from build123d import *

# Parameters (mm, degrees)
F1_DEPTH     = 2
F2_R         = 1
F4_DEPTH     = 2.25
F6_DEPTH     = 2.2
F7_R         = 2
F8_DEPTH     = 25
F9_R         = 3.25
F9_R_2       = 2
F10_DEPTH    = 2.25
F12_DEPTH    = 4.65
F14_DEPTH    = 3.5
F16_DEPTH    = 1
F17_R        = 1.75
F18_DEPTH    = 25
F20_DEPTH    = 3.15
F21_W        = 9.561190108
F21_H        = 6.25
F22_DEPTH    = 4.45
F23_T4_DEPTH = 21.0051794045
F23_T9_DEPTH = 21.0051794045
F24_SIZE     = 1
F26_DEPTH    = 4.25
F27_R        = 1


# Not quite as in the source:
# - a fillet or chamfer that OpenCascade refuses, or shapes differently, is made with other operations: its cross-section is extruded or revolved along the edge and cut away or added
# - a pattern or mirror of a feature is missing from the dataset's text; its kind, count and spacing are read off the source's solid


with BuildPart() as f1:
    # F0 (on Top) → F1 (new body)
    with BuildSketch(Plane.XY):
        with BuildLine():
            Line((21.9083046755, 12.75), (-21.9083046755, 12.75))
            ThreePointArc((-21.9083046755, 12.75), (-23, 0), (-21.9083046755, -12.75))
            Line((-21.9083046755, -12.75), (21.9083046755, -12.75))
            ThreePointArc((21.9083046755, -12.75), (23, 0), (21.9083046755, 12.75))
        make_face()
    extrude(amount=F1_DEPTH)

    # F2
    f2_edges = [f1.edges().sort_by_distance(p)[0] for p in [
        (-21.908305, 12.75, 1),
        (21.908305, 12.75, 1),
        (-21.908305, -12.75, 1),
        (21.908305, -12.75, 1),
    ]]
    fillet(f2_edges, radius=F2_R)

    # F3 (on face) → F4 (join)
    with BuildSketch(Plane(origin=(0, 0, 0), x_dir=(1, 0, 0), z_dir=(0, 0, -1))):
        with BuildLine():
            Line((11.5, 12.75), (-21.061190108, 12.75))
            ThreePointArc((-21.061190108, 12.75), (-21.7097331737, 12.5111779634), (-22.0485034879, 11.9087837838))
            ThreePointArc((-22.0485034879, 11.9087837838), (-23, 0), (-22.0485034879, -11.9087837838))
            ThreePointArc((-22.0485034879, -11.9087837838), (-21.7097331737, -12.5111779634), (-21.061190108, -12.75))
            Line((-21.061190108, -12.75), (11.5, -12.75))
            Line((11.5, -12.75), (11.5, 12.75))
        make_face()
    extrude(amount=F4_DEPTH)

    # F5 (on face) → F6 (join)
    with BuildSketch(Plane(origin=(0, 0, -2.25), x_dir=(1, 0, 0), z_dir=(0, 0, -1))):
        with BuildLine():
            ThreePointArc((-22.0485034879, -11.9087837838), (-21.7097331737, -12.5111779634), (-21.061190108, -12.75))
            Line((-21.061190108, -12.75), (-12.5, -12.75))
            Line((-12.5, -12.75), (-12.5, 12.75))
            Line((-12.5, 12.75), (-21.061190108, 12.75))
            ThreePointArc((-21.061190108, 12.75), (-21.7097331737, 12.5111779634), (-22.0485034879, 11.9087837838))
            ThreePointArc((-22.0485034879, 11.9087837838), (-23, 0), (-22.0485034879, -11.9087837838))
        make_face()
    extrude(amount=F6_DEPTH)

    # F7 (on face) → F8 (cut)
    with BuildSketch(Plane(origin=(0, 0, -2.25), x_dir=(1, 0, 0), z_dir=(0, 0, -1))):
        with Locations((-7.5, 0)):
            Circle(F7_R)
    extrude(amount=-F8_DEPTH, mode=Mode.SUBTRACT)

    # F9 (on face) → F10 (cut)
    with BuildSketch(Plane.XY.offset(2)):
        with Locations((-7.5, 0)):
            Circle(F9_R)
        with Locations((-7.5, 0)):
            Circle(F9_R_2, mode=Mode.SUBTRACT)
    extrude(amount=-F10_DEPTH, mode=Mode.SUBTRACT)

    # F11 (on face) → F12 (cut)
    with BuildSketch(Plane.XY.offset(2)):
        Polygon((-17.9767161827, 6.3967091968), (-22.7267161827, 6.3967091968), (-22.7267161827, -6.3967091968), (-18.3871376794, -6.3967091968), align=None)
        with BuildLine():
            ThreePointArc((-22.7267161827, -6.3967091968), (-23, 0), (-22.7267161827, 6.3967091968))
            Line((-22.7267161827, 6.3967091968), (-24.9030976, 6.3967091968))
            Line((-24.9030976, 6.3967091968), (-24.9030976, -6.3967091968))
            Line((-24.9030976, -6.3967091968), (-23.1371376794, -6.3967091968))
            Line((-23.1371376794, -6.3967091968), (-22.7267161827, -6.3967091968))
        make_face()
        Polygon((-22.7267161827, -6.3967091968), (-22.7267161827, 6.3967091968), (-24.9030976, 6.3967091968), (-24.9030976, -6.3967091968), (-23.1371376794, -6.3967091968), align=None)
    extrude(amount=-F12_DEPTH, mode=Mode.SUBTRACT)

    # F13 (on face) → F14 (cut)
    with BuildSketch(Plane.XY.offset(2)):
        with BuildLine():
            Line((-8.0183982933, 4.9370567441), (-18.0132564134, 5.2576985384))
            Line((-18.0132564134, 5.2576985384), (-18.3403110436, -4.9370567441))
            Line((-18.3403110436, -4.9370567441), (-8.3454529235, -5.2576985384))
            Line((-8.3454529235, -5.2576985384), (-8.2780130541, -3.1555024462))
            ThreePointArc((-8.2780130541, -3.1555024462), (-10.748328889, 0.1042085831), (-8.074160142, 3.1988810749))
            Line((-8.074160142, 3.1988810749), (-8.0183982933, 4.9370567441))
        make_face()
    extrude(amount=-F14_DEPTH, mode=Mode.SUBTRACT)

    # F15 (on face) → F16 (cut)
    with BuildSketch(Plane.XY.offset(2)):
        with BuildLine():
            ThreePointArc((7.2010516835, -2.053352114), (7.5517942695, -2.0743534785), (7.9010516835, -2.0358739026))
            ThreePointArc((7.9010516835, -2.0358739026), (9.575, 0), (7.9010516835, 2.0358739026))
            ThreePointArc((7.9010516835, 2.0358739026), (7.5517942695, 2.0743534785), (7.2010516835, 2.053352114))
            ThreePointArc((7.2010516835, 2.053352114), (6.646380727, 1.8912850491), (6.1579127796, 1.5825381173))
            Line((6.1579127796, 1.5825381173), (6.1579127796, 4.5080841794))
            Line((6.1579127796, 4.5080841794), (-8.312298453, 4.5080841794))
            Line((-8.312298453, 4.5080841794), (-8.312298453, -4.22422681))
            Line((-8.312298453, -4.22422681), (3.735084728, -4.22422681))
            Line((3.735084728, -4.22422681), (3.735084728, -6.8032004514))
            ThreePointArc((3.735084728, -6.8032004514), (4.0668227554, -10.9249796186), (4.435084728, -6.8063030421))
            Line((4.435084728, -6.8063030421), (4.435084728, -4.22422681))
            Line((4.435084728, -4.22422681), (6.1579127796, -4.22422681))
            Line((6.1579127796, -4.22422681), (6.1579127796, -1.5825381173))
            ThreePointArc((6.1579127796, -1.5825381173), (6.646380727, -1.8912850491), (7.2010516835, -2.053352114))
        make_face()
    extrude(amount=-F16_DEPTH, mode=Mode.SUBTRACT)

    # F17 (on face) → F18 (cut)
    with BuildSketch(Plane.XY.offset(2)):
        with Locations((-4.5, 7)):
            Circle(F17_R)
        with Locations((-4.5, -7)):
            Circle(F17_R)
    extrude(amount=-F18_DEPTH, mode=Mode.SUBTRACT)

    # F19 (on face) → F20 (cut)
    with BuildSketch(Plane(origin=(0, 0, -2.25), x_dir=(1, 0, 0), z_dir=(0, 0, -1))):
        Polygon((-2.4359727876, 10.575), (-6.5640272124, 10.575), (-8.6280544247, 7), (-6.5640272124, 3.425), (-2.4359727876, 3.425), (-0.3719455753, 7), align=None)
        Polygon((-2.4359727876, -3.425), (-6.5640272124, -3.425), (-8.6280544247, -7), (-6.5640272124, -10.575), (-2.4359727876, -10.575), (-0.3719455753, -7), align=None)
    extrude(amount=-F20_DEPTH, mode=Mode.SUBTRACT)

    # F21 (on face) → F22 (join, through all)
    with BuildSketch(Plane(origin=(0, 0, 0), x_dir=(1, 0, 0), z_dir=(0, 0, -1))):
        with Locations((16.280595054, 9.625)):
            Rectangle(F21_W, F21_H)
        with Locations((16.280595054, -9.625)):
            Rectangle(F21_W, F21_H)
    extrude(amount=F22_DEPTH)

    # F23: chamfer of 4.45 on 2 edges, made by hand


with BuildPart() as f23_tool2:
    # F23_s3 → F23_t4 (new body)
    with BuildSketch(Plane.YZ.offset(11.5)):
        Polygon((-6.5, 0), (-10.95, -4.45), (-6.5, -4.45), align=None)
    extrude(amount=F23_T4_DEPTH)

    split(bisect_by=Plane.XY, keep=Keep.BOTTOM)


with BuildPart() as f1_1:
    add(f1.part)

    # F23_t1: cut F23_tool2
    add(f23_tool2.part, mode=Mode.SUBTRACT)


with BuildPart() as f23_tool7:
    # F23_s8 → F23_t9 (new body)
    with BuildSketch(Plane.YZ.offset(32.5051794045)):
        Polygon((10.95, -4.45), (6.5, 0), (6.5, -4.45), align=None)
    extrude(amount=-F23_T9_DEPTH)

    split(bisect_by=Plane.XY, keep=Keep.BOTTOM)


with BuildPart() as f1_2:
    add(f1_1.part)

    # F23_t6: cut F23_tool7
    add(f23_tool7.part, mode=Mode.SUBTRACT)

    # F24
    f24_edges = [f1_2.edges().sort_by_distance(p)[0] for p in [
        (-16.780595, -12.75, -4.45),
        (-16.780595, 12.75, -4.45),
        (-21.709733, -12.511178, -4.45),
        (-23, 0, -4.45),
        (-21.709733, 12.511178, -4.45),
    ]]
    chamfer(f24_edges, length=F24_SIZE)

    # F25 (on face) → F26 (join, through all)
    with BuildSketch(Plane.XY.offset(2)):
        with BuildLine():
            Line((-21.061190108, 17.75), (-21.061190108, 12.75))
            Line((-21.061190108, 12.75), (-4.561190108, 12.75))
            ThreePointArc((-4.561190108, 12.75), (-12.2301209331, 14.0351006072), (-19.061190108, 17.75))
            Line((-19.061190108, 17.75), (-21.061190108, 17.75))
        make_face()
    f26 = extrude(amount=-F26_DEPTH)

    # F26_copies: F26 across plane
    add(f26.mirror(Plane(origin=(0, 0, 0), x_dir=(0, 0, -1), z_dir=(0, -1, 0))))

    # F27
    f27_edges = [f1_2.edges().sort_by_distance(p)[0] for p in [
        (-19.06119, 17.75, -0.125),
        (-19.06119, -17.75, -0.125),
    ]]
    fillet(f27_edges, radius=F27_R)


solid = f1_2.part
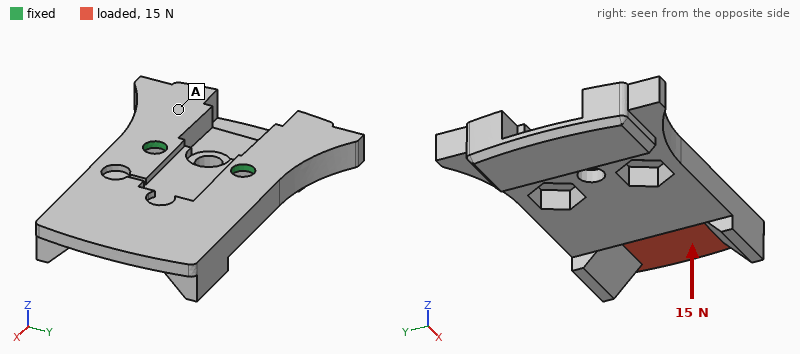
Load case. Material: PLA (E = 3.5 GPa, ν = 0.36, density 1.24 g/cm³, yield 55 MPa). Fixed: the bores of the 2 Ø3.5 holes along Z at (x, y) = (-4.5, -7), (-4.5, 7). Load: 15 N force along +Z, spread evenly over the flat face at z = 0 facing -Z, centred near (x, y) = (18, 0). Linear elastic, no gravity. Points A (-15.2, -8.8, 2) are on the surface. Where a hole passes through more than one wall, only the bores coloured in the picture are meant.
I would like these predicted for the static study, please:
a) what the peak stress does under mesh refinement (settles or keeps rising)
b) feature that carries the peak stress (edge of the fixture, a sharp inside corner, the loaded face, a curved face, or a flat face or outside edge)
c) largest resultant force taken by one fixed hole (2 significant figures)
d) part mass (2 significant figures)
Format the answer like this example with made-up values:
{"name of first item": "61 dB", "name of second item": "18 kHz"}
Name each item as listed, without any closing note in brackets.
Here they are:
{"what the peak stress does under mesh refinement": "keeps rising", "feature that carries the peak stress": "edge of the fixture", "largest resultant force taken by one fixed hole": "8.1 N", "part mass": "5.3 g"}
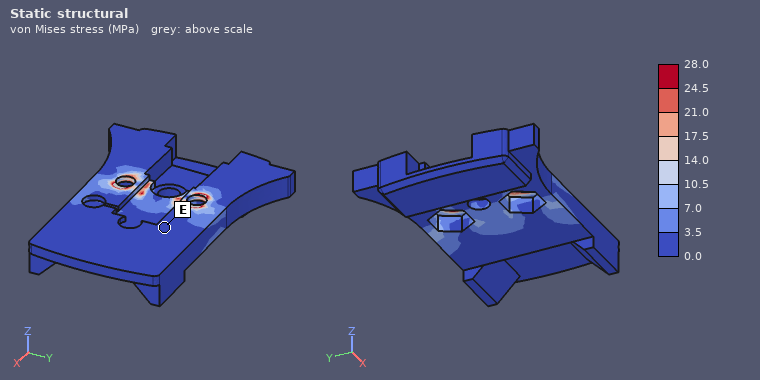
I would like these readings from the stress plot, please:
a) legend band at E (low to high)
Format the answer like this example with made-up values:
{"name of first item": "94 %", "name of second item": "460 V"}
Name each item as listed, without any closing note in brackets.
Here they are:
{"legend band at E": "0.0 to 3.5 MPa"}
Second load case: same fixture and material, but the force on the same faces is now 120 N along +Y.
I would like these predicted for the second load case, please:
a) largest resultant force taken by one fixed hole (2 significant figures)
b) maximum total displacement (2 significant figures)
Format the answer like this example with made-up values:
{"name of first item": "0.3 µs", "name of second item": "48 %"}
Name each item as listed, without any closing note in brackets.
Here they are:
{"largest resultant force taken by one fixed hole": "170 N", "maximum total displacement": "0.17 mm"}
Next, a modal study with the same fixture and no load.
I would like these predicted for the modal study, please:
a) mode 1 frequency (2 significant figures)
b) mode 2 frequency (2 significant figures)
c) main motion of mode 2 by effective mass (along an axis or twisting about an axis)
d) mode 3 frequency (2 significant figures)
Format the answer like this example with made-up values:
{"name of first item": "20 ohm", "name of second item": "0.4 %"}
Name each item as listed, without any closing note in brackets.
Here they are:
{"mode 1 frequency": "750 Hz", "mode 2 frequency": "1900 Hz", "main motion of mode 2 by effective mass": "along Z", "mode 3 frequency": "2100 Hz"}
